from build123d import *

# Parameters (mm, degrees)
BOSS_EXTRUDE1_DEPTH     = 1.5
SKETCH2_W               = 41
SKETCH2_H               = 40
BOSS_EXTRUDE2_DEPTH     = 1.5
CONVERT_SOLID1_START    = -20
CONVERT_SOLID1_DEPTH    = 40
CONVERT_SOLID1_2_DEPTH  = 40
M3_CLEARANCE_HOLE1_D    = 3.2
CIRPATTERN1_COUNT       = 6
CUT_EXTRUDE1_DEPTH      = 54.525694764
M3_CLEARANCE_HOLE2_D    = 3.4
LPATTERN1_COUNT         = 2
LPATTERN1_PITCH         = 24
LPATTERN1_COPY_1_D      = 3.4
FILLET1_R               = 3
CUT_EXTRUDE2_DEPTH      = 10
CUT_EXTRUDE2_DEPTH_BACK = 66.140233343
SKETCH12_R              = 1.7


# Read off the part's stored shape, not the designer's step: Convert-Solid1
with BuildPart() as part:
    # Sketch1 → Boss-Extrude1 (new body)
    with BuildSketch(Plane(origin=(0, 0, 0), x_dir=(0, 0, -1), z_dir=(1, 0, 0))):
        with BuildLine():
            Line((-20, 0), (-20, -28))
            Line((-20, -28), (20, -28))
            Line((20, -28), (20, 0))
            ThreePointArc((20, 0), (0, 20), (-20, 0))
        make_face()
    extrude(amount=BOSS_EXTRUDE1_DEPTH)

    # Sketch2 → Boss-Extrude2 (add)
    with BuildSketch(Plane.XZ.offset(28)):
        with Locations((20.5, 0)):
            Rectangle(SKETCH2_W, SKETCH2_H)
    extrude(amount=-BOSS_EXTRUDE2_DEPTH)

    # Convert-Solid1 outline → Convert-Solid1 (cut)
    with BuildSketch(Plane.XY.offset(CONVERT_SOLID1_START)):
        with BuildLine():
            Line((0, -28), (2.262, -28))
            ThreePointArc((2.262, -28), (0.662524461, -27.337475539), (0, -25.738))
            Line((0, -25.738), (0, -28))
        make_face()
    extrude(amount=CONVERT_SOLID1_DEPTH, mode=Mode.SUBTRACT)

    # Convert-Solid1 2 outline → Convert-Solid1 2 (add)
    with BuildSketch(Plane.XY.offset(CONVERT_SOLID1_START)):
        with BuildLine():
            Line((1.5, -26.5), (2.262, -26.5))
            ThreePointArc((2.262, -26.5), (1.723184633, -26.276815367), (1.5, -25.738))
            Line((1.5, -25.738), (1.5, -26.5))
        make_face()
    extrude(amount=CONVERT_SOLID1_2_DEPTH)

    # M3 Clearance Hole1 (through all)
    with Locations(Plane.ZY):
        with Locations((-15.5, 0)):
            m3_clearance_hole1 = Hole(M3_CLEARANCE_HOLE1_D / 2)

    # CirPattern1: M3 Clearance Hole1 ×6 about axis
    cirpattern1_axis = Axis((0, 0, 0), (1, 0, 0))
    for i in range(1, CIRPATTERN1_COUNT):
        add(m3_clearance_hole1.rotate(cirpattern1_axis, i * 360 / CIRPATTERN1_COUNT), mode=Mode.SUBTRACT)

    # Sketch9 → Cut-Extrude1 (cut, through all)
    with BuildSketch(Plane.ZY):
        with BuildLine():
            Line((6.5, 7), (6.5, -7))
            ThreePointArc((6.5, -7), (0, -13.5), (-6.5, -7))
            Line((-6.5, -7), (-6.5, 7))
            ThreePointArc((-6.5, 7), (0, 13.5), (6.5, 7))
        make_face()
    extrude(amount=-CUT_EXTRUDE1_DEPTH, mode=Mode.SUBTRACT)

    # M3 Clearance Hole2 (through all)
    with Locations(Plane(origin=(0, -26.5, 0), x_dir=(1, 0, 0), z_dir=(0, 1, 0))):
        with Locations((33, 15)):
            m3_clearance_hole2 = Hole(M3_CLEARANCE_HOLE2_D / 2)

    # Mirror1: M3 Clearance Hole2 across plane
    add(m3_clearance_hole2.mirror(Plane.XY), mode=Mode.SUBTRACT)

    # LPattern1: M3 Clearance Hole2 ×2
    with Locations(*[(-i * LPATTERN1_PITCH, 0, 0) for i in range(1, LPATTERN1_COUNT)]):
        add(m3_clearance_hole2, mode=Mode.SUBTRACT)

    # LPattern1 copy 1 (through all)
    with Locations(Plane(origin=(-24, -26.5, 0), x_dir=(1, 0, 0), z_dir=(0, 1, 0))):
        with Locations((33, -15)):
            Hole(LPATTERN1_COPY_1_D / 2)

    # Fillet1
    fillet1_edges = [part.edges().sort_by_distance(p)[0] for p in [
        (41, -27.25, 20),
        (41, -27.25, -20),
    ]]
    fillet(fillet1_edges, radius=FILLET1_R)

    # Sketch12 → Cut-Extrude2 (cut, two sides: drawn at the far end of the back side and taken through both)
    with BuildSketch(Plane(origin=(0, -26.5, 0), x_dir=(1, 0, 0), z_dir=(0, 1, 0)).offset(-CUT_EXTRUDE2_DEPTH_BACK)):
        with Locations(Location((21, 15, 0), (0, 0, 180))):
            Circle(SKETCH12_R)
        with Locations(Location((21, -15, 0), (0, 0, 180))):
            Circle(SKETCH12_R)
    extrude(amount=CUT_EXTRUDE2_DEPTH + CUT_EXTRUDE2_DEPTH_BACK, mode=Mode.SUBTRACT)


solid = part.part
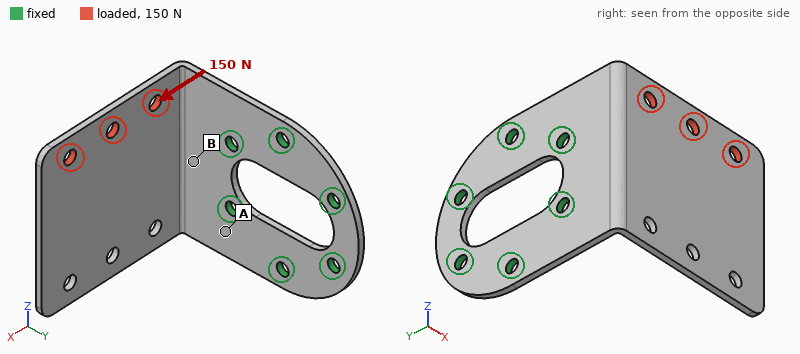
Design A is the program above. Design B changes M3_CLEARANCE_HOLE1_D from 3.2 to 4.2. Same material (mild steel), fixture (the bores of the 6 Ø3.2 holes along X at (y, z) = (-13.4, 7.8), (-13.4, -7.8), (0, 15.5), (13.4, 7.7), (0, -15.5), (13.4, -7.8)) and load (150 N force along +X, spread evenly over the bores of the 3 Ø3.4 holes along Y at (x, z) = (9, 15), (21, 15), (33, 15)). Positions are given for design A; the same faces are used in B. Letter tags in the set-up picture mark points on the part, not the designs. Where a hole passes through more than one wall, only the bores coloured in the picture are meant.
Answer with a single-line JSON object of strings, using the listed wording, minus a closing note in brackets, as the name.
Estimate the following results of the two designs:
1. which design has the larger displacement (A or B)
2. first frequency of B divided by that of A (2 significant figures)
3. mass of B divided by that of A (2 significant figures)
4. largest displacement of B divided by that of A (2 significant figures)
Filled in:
{"which design has the larger displacement": "A", "first frequency of B divided by that of A": "1.0", "mass of B divided by that of A": "0.99", "largest displacement of B divided by that of A": "0.91"}
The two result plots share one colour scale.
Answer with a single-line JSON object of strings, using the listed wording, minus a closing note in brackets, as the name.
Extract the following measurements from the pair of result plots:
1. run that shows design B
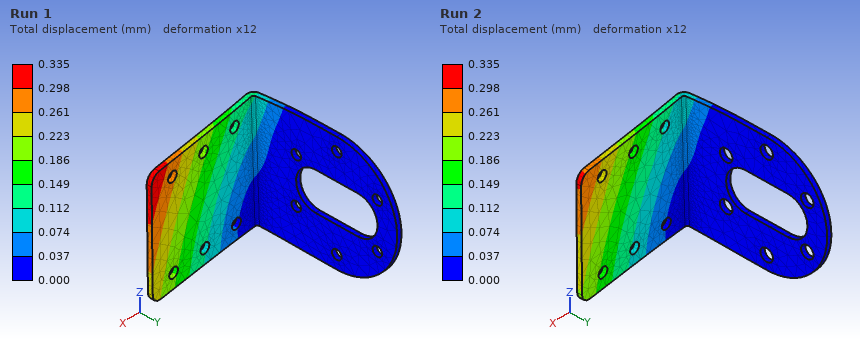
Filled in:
{"run that shows design B": "Run 2"}
